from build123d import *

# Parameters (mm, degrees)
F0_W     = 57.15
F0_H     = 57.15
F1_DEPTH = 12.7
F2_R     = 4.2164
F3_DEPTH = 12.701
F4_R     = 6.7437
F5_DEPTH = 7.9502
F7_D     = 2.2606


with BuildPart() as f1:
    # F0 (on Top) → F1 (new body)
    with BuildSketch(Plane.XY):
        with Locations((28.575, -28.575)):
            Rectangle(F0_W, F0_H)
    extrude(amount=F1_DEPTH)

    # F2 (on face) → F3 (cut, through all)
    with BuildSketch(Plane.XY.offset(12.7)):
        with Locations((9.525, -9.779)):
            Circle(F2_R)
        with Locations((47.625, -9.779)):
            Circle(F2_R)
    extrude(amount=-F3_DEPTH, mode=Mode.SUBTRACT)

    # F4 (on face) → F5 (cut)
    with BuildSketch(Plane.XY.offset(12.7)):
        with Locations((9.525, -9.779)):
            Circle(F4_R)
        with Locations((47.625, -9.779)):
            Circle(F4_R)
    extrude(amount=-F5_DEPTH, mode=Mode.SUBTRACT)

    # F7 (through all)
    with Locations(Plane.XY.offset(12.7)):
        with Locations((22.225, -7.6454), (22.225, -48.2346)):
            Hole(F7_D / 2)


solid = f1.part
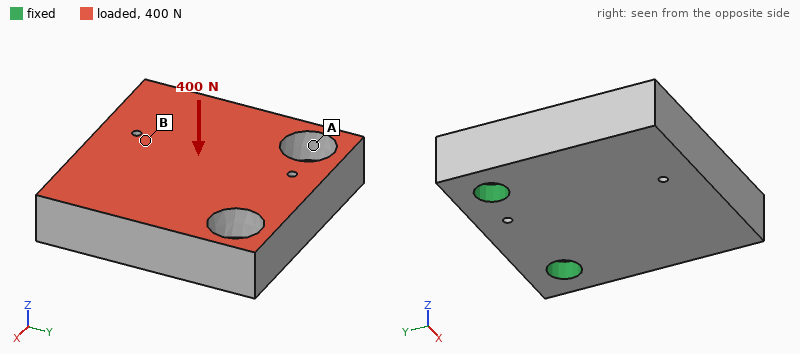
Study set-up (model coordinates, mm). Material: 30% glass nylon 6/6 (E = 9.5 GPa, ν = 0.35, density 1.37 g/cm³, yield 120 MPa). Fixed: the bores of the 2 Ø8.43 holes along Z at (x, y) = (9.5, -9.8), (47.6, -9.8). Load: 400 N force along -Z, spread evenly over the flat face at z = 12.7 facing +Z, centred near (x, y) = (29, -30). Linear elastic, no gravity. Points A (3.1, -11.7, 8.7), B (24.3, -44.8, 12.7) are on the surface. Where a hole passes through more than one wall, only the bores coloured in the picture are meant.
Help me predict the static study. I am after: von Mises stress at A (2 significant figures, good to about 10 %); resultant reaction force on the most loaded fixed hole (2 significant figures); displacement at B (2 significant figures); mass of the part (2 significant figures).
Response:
8.0 MPa
210 N
0.12 mm
53 g
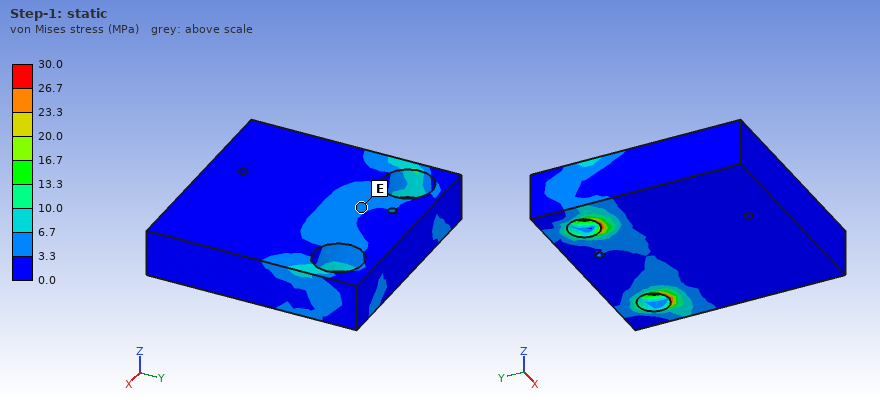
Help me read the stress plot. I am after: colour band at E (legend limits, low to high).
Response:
3.3 to 6.7 MPa
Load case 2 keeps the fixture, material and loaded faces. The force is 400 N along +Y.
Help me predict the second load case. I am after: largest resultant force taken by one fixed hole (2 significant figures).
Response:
200 N
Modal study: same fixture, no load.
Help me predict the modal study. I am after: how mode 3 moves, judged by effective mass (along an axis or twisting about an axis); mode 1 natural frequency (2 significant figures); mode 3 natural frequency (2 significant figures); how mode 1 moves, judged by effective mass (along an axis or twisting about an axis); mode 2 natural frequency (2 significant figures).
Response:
along X
1300 Hz
5100 Hz
along Z
3700 Hz
